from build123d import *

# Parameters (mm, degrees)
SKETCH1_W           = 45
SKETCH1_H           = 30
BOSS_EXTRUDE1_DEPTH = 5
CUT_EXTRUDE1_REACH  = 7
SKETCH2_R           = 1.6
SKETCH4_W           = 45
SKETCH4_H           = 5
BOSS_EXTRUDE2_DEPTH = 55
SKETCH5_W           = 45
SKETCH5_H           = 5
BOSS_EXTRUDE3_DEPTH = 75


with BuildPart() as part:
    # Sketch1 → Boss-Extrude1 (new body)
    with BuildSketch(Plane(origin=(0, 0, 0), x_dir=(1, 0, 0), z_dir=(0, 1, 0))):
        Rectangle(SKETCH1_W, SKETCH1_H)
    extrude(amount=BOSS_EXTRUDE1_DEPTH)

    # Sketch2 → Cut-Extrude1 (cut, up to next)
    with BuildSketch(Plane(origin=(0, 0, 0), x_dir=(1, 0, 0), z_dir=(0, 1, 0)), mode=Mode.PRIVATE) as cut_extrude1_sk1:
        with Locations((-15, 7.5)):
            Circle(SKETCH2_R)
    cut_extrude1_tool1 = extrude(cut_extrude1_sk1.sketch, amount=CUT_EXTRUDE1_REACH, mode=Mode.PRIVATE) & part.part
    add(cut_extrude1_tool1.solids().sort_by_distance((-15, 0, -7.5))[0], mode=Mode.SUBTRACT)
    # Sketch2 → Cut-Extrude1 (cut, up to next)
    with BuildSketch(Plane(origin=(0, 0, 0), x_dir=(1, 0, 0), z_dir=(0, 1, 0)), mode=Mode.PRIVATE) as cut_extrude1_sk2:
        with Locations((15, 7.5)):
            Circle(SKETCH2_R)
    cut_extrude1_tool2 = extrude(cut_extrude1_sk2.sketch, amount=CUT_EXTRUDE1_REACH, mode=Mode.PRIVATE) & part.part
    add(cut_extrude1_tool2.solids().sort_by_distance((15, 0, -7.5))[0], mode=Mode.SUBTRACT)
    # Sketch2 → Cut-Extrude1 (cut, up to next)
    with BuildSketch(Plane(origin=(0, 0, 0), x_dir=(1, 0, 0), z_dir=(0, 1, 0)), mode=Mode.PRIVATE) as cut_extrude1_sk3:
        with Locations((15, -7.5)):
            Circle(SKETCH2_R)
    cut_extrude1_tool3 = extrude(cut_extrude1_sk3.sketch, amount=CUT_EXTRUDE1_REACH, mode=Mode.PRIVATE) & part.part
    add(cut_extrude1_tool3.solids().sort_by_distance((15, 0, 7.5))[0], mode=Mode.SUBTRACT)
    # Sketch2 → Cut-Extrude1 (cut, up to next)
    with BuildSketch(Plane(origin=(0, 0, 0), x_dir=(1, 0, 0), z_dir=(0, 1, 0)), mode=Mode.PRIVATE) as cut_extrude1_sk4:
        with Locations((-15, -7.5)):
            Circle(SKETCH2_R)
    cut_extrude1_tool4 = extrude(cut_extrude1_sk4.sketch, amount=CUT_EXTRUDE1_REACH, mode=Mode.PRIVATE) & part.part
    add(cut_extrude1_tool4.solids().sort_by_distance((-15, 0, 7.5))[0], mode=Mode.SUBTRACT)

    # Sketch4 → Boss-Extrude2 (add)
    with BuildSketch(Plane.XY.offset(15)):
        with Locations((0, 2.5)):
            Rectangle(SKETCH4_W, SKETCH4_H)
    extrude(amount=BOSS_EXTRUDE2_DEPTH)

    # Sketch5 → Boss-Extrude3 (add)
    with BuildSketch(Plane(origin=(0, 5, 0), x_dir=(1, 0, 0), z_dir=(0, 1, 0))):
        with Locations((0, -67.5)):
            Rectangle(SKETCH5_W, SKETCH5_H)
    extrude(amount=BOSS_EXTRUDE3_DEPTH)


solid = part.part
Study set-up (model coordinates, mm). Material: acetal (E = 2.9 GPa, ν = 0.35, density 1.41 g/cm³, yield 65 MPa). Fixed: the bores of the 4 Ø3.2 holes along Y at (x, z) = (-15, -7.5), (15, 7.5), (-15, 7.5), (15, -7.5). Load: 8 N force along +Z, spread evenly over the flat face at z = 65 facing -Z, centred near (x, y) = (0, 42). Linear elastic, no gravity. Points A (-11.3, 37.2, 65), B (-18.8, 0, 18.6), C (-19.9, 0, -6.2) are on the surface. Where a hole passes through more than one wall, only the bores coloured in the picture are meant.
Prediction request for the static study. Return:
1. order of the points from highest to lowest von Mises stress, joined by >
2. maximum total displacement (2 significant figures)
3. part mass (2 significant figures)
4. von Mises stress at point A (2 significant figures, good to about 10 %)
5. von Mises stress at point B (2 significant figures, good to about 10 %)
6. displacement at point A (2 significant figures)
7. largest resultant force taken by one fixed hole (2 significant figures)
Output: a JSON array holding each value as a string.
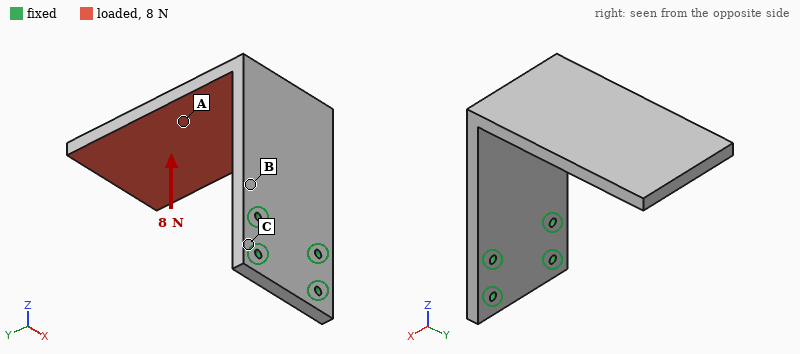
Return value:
["B > A > C", "1.4 mm", "51 g", "0.51 MPa", "1.7 MPa", "0.68 mm", "5.5 N"]
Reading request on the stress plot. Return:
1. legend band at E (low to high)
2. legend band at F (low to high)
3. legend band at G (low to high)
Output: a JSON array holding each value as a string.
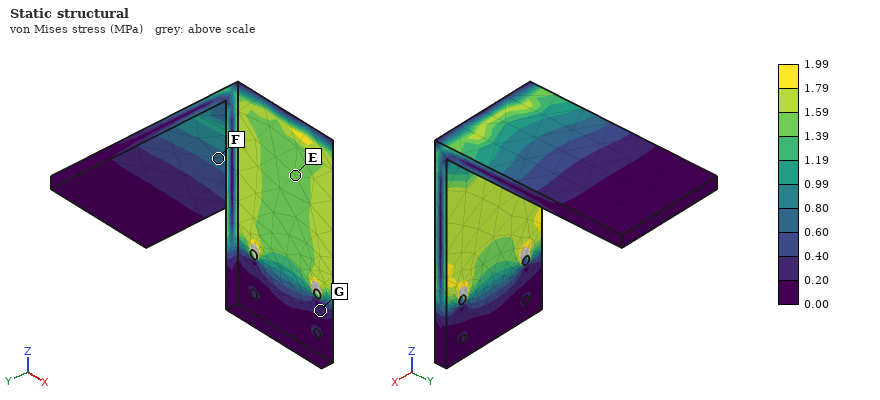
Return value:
["1.39 to 1.59 MPa", "0.60 to 0.80 MPa", "0.20 to 0.40 MPa"]
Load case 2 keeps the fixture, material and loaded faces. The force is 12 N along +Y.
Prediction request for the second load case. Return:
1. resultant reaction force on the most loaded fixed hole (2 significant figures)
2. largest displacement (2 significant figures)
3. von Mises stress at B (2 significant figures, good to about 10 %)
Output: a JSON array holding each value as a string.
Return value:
["15 N", "1.3 mm", "3.1 MPa"]
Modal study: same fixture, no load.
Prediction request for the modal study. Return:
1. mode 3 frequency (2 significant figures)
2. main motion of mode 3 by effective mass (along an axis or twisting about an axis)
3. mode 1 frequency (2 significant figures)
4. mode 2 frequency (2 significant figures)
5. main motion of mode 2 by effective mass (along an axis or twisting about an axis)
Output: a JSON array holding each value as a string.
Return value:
["230 Hz", "along Y", "82 Hz", "140 Hz", "along X"]
